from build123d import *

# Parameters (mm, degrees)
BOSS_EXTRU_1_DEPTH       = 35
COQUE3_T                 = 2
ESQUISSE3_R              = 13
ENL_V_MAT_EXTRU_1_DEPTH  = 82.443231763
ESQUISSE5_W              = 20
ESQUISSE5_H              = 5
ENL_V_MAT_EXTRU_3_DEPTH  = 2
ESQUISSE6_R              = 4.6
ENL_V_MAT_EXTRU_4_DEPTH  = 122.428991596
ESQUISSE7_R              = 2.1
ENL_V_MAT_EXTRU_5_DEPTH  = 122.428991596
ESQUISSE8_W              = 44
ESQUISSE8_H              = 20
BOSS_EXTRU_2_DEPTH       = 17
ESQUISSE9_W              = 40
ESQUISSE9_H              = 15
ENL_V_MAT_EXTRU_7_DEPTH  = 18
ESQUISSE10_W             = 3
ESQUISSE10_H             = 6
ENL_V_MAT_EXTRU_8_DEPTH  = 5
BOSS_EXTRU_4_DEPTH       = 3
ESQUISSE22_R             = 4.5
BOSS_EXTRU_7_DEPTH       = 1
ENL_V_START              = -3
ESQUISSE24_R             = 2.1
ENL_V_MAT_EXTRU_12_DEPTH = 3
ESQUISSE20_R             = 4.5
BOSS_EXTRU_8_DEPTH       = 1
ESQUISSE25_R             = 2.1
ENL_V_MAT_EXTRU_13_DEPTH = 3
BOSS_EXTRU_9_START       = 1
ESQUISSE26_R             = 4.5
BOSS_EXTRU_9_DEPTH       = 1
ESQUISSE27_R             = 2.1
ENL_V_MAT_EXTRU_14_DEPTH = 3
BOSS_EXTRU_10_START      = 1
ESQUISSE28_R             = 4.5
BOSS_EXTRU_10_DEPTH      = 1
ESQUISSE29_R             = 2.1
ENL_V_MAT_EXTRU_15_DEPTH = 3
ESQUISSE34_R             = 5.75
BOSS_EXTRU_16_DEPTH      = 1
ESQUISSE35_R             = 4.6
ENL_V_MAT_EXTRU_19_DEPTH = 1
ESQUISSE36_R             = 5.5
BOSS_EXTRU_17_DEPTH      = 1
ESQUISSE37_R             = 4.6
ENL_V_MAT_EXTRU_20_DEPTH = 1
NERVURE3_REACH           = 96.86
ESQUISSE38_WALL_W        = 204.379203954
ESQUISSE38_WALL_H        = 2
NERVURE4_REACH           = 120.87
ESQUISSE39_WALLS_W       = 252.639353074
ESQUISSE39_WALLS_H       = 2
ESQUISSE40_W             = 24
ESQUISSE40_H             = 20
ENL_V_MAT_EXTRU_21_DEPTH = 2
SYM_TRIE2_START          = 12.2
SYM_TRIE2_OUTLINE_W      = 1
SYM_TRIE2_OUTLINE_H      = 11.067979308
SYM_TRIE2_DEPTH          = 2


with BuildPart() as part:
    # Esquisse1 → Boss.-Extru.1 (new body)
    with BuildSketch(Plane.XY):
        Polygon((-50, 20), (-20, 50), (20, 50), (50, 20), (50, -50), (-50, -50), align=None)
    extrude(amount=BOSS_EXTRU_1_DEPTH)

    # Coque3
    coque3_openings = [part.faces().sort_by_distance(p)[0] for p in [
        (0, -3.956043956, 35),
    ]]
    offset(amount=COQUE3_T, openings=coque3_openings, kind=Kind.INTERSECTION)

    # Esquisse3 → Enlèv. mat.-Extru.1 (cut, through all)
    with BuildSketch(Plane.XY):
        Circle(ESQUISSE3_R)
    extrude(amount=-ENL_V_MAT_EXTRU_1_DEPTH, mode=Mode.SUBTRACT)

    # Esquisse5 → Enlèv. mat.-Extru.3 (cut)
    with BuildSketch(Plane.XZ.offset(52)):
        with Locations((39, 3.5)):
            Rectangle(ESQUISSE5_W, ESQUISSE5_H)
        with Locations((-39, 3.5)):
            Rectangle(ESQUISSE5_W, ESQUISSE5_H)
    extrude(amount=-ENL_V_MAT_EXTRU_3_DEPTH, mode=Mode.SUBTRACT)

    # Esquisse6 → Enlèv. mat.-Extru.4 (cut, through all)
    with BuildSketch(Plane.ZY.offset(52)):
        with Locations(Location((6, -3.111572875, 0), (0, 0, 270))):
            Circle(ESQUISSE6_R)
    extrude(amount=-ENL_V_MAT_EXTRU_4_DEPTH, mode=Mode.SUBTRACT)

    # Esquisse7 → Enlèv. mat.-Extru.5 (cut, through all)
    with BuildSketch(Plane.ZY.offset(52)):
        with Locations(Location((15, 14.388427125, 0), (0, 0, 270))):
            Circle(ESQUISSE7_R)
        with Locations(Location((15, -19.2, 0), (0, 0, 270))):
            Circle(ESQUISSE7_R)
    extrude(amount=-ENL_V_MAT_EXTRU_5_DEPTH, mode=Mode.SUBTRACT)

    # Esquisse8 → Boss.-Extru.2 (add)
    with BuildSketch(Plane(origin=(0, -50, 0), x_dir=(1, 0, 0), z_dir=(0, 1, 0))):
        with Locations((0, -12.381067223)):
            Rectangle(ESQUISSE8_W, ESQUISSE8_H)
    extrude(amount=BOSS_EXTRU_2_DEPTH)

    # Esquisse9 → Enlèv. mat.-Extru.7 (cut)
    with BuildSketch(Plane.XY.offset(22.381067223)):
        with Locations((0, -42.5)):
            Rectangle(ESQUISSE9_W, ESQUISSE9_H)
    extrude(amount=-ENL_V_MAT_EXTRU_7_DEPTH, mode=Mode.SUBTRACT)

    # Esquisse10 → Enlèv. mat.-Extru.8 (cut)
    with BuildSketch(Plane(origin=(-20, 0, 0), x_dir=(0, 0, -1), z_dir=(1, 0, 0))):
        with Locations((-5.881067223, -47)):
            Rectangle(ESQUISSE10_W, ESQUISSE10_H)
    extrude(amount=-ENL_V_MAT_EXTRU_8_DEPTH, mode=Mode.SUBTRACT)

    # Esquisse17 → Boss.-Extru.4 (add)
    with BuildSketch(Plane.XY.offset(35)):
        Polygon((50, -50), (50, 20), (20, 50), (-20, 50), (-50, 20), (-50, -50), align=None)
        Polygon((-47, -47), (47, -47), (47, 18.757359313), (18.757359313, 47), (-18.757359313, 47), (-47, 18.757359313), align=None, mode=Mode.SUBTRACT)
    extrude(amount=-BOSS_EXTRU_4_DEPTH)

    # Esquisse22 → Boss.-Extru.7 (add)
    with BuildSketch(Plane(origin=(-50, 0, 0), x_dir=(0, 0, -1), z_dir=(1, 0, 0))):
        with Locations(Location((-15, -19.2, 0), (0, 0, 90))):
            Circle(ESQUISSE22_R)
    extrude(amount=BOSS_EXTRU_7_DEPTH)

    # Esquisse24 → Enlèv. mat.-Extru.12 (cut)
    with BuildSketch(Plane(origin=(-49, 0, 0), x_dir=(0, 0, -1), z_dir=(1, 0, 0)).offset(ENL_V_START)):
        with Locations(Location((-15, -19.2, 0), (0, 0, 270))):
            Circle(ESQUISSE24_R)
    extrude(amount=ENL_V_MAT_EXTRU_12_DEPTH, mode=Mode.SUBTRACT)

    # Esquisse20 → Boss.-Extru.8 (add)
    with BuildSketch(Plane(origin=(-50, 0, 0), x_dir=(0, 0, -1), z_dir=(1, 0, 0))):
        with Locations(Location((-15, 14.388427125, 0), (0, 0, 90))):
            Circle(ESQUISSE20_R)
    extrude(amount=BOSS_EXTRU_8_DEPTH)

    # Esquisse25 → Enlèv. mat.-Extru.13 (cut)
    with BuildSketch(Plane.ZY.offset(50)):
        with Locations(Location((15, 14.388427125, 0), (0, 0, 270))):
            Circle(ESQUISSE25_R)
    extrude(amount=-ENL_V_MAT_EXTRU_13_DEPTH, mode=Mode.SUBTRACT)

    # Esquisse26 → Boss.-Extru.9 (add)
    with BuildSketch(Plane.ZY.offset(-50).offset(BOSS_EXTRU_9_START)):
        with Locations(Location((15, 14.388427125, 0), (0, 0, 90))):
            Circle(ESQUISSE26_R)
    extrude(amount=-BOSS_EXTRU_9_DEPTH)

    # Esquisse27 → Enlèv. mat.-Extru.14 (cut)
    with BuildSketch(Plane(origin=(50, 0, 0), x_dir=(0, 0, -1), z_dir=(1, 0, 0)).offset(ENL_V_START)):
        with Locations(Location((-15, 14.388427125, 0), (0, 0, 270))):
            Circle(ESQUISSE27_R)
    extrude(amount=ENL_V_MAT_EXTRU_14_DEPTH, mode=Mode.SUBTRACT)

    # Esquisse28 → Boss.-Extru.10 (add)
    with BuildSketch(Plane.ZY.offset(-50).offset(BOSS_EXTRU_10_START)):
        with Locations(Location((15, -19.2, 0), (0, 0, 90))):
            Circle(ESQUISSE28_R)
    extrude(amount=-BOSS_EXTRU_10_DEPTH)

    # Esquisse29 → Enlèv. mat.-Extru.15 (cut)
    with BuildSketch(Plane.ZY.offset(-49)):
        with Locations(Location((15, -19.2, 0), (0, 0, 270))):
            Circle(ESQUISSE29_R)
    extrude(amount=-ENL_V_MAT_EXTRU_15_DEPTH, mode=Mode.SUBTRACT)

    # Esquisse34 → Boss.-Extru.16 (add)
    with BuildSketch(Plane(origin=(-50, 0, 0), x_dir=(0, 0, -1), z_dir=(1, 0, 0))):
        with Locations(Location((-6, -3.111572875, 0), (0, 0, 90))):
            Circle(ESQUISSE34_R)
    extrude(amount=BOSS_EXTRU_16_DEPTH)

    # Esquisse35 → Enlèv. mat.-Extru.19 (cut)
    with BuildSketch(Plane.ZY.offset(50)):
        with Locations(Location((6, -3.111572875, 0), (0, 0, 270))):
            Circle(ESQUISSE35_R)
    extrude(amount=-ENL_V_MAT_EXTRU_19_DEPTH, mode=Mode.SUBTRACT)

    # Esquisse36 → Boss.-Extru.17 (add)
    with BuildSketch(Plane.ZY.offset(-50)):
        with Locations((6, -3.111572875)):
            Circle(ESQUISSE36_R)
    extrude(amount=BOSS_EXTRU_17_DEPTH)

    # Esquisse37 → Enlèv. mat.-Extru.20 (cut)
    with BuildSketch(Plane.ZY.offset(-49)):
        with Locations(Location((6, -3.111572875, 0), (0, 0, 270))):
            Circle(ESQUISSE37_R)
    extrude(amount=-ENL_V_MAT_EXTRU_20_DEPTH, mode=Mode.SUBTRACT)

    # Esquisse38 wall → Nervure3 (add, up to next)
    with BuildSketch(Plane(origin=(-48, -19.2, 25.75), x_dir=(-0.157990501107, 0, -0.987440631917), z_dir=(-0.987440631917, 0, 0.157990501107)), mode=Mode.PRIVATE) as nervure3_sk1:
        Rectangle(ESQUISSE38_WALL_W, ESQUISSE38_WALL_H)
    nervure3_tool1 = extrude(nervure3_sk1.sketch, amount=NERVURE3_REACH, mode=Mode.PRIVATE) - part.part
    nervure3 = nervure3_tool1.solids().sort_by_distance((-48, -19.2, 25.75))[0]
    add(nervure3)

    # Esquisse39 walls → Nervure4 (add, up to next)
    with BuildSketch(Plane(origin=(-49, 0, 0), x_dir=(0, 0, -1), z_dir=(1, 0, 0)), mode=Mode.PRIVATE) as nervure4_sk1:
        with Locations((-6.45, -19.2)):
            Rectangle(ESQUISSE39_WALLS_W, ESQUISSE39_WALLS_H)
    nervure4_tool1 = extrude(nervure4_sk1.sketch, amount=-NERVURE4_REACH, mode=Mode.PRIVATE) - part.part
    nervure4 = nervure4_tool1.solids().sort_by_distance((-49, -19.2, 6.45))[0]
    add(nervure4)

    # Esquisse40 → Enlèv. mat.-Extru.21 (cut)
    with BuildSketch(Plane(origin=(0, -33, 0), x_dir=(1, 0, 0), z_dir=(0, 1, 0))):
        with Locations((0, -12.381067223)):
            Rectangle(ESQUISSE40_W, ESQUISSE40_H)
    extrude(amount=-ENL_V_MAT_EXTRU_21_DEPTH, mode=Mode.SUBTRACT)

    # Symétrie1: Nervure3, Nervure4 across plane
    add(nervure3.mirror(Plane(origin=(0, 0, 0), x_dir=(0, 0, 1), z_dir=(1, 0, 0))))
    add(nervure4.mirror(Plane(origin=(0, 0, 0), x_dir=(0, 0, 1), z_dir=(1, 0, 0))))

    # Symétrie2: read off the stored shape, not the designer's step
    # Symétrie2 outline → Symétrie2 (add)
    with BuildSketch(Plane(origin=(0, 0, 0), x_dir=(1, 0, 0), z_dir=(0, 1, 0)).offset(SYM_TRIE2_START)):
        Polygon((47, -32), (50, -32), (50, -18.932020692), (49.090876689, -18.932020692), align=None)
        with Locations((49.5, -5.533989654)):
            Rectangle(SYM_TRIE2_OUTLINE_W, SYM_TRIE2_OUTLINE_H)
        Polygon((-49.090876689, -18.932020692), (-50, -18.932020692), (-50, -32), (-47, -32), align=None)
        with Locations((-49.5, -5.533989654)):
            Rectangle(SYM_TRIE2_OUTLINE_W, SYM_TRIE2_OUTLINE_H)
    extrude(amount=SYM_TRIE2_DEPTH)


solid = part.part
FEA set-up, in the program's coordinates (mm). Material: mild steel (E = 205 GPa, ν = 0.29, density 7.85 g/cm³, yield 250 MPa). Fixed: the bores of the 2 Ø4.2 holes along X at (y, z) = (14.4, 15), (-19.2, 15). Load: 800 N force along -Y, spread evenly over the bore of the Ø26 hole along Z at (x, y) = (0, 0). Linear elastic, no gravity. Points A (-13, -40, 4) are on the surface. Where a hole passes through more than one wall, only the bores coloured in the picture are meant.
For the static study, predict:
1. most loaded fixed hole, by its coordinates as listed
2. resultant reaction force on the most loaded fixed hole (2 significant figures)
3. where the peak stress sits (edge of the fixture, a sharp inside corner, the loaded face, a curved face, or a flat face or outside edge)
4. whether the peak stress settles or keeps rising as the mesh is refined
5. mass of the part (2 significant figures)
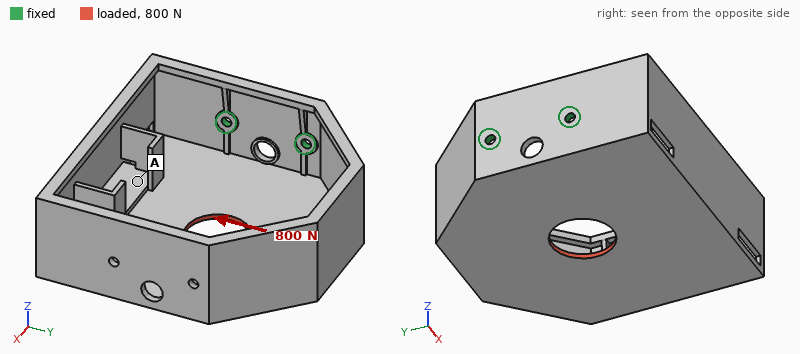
(-19.2, 15)
1.2 kN
edge of the fixture
keeps rising
400 g
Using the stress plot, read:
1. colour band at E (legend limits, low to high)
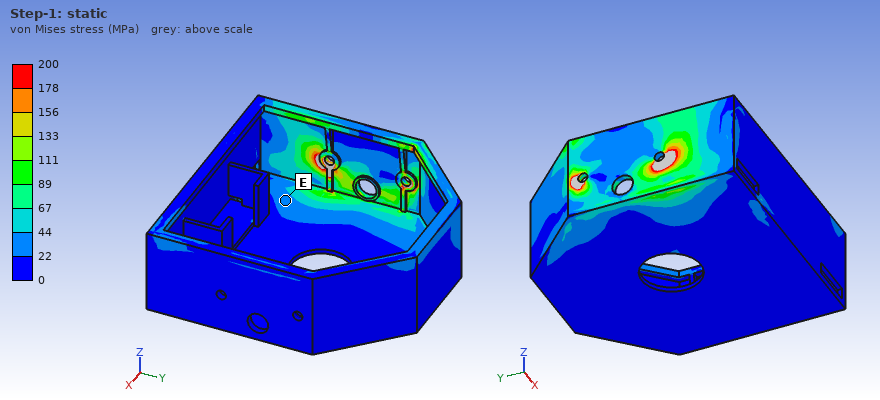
22 to 44 MPa
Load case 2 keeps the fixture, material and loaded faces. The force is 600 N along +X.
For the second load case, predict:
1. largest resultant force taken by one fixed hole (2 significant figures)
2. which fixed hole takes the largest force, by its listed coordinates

360 N
(14.4, 15)
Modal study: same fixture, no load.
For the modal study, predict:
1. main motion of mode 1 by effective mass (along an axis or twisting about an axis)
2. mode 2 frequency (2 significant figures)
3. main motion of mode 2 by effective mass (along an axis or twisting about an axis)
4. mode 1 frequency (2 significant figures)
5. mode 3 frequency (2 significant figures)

along Z
340 Hz
along Y
190 Hz
730 Hz
